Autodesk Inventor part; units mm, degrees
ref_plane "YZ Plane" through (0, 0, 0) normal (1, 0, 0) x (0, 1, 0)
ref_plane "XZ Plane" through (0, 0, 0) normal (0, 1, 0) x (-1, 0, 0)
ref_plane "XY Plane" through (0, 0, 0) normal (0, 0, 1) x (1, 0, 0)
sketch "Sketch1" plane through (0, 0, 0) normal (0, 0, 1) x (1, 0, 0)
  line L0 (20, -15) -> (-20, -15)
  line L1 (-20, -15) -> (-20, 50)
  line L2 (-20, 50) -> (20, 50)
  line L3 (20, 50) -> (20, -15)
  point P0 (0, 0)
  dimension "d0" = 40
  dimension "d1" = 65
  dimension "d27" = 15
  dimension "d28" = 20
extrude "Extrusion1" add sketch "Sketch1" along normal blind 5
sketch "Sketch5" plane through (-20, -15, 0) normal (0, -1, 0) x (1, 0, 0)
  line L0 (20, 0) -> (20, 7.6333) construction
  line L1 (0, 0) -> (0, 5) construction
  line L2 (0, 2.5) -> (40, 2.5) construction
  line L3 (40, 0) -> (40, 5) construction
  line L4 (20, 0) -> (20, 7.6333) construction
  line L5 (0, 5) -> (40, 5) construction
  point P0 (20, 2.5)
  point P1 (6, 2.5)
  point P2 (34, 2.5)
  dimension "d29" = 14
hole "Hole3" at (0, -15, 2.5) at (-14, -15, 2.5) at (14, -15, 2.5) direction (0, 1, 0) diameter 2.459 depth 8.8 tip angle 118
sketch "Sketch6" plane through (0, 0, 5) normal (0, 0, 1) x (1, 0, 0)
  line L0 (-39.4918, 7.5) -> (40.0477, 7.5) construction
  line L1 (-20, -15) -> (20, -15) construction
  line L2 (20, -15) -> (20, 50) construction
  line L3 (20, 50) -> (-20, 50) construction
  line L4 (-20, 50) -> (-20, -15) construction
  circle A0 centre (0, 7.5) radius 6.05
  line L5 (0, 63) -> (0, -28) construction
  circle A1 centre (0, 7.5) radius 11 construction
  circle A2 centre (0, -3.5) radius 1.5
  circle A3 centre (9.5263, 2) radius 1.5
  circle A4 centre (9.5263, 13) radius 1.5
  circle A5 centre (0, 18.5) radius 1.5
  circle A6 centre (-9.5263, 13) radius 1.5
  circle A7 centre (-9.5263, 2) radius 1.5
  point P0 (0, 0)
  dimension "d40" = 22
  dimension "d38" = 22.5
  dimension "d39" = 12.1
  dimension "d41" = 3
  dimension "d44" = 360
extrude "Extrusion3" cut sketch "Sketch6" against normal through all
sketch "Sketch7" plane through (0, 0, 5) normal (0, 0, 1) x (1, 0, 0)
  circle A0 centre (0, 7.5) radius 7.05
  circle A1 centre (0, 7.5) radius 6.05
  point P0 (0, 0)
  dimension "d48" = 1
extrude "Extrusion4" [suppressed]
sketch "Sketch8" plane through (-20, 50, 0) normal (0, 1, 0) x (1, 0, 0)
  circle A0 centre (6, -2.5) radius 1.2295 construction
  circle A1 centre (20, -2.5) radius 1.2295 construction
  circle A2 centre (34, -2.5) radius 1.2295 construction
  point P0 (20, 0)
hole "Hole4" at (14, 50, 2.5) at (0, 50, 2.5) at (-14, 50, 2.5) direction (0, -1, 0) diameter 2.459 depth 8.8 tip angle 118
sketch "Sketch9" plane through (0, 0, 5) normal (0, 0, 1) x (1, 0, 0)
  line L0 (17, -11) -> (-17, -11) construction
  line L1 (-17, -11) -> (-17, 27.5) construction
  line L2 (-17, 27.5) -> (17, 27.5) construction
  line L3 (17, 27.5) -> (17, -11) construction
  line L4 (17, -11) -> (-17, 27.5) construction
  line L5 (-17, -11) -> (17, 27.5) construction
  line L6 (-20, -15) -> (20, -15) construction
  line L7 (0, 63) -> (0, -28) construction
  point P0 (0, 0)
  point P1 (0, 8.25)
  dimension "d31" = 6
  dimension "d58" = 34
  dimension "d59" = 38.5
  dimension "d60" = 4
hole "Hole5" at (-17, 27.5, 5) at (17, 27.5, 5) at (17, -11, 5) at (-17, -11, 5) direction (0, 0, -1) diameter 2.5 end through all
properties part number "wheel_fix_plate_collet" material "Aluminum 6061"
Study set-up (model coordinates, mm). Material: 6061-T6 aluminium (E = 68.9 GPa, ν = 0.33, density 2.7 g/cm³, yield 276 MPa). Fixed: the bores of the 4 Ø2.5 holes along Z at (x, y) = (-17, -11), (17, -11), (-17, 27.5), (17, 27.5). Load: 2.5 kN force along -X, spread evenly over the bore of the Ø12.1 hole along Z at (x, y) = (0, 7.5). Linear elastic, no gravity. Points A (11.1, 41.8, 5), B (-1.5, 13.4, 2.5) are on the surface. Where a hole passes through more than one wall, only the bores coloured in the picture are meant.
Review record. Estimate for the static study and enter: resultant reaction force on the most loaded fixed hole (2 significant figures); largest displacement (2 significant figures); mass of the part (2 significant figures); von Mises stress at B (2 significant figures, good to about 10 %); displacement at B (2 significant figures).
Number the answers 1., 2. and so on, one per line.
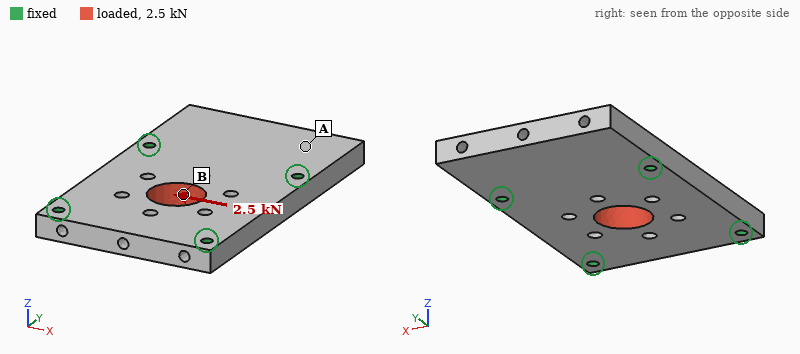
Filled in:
1. 740 N
2. 7.2 µm
3. 32 g
4. 25 MPa
5. 5.9 µm
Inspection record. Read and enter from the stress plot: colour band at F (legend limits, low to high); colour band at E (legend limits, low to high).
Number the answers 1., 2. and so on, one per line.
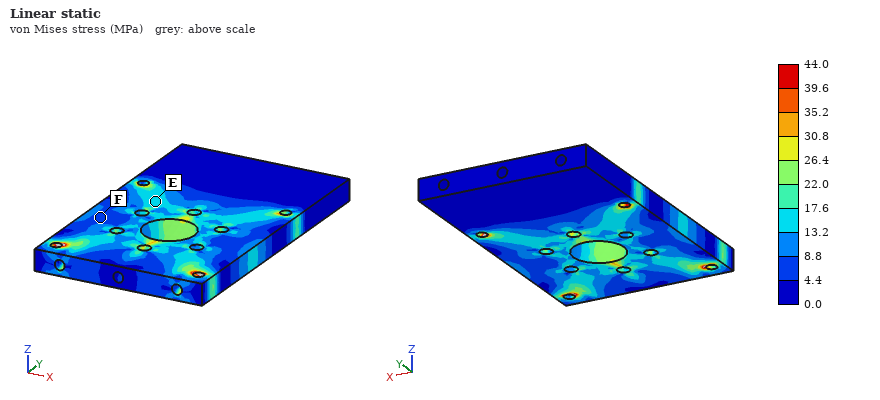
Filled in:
1. 4.4 to 8.8 MPa
2. 13.2 to 17.6 MPa
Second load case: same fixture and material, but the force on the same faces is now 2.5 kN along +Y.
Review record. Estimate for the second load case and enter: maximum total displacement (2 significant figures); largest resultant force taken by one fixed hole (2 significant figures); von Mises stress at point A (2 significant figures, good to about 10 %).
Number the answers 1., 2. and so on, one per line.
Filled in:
1. 6.0 µm
2. 730 N
3. 3.0 MPa
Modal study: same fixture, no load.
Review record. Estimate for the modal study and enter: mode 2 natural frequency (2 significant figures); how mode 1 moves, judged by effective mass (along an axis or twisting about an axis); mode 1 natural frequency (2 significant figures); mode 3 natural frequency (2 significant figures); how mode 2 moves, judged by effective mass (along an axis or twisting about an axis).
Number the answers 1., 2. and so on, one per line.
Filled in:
1. 11 kHz
2. along Z
3. 6300 Hz
4. 12 kHz
5. along Z
